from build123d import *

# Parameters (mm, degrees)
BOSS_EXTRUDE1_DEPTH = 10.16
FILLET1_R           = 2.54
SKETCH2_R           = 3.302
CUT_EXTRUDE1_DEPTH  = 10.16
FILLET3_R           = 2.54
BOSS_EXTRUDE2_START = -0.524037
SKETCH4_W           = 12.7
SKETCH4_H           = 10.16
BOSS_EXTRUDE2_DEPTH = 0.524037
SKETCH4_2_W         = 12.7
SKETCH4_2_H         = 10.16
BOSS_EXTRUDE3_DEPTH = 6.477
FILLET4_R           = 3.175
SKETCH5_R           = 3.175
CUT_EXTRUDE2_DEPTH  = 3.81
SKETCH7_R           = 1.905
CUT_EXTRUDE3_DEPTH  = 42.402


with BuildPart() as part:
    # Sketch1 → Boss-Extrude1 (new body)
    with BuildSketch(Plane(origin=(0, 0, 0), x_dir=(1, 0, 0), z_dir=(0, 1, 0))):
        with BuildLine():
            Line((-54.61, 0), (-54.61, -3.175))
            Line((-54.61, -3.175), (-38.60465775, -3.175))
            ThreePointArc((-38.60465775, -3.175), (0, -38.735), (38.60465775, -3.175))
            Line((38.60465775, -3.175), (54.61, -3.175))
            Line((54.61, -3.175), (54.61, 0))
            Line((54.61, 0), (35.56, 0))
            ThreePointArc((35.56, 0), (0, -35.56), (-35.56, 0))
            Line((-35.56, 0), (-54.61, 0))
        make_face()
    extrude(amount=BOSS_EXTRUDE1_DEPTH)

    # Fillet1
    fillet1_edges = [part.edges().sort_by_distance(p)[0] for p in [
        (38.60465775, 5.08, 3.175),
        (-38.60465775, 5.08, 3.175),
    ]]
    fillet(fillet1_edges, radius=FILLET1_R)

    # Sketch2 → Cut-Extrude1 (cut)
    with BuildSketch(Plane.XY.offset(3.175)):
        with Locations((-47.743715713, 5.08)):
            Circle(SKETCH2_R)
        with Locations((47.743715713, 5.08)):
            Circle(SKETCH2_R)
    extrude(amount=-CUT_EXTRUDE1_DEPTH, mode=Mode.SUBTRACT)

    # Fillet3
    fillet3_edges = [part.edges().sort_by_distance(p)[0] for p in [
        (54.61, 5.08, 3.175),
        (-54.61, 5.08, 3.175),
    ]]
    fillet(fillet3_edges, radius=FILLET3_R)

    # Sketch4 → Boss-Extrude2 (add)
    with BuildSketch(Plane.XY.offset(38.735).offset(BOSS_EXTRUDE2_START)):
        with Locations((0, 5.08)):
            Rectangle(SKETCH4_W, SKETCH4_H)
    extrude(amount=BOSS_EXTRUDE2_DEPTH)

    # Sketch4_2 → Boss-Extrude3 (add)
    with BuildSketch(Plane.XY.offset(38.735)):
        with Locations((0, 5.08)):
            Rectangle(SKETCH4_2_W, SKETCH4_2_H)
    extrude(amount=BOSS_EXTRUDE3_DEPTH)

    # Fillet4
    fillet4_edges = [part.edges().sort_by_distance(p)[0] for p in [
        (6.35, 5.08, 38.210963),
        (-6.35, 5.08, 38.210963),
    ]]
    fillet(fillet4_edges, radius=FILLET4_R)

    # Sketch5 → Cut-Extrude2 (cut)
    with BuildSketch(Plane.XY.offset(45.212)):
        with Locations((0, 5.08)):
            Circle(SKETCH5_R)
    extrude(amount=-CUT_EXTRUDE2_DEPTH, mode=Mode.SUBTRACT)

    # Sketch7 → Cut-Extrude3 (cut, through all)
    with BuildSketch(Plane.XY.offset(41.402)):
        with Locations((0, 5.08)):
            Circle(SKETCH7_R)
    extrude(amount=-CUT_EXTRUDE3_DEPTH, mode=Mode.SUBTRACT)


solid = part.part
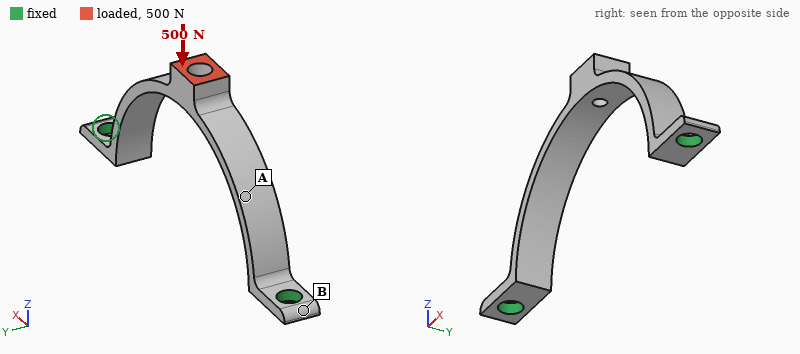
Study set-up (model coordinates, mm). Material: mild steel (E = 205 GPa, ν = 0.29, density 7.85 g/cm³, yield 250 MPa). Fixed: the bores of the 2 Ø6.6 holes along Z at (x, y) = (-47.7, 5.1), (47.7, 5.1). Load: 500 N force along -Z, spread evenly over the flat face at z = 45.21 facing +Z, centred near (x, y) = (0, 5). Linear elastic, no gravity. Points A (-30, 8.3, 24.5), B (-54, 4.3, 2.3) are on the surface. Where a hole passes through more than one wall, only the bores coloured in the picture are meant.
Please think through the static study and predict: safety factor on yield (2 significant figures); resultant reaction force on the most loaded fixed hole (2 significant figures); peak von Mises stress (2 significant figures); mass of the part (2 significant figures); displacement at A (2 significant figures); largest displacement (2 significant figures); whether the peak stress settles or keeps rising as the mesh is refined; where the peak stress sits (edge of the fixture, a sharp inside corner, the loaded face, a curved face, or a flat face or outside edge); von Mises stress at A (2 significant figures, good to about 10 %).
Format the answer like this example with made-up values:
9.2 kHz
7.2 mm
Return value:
2.3
330 N
110 MPa
41 g
19 µm
31 µm
settles
a curved face
44 MPa
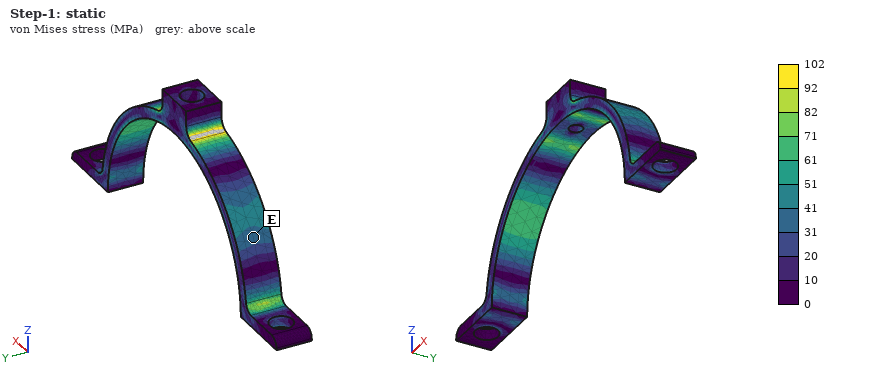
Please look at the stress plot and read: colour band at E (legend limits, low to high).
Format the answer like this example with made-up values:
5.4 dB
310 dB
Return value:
31 to 41 MPa
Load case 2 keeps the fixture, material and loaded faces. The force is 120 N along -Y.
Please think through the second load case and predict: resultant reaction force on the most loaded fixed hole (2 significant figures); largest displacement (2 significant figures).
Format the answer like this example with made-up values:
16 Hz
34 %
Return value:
60 N
0.14 mm
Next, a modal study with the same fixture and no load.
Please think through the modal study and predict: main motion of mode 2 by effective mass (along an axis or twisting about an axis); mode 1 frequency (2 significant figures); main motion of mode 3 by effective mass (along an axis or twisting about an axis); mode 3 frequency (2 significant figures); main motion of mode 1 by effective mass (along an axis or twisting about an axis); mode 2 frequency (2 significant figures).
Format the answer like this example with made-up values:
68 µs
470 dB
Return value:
along X
1400 Hz
twisting about Z
4700 Hz
along Y
2100 Hz
